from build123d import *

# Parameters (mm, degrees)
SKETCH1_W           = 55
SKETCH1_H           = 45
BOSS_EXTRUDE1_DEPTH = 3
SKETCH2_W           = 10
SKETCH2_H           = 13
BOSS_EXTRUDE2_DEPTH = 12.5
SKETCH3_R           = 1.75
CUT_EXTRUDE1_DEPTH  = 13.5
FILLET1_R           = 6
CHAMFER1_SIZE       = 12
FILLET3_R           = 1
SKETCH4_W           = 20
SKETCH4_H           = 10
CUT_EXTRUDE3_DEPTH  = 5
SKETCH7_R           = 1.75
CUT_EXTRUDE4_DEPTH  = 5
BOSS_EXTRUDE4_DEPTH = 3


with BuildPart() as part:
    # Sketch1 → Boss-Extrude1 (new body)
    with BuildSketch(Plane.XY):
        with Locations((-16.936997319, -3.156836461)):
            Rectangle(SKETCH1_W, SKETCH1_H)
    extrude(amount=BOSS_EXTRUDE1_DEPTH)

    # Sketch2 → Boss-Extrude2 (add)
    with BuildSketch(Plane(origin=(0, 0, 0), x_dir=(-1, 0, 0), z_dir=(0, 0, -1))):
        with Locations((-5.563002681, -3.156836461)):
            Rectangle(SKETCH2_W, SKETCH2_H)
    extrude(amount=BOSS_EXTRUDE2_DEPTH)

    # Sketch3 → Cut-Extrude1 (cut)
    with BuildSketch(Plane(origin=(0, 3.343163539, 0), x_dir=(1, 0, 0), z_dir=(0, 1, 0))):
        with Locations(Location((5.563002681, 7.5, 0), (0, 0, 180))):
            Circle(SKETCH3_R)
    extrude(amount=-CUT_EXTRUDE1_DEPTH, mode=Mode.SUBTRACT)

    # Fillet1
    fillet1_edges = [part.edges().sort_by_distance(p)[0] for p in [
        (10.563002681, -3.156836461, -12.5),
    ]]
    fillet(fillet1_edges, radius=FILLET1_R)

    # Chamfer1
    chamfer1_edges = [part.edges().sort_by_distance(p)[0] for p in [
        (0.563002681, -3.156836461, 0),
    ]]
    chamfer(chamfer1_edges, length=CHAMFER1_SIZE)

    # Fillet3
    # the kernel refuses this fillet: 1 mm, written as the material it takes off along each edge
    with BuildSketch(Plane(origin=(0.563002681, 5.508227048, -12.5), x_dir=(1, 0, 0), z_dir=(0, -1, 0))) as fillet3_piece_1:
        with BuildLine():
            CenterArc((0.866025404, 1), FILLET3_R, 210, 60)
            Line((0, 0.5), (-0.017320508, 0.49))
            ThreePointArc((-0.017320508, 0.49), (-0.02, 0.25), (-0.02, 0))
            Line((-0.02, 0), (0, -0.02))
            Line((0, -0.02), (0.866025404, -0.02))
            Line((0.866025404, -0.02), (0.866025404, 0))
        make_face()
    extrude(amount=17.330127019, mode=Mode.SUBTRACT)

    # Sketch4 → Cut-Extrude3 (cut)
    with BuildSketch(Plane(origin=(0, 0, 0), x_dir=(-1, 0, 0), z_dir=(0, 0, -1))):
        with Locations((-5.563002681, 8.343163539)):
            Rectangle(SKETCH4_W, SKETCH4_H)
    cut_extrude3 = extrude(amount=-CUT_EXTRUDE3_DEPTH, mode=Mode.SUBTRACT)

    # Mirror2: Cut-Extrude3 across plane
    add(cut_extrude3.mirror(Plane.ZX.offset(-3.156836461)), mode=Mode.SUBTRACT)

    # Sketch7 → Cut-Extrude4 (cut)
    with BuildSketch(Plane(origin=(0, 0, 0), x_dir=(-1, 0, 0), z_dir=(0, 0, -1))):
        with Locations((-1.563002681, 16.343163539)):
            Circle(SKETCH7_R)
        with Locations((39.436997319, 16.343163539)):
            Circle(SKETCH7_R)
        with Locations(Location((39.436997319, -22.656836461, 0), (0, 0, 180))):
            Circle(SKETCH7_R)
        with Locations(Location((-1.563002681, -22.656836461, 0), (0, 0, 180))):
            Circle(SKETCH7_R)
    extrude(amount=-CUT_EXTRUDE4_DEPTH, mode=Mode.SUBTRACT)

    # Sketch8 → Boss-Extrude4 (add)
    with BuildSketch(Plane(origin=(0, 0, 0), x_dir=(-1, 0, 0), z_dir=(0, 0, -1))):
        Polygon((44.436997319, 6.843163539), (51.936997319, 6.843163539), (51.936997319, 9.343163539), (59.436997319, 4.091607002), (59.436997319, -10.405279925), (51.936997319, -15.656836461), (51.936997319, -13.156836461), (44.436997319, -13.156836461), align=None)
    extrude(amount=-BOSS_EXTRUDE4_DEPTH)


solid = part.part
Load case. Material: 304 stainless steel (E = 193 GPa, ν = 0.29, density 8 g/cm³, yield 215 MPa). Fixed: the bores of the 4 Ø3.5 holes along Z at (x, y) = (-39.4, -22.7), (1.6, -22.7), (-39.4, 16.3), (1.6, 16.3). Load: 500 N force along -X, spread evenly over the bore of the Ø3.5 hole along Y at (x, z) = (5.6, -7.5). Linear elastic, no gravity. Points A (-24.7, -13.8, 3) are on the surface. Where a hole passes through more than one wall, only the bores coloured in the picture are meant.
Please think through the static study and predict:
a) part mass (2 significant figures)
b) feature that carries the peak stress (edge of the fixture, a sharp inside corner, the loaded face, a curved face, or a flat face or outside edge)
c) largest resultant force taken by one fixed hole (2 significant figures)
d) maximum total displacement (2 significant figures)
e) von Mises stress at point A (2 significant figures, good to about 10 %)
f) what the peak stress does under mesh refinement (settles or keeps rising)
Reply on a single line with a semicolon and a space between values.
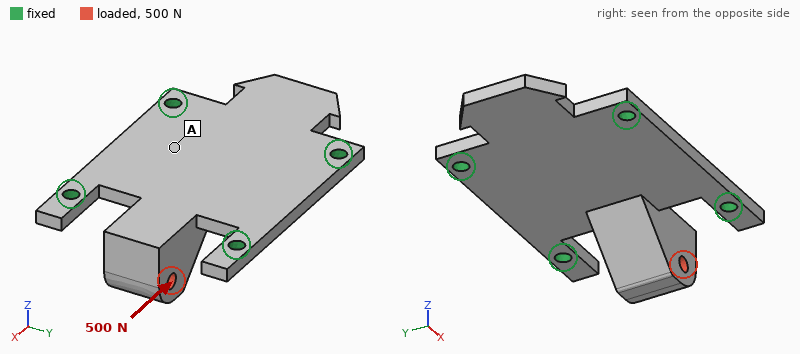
77 g; a sharp inside corner; 200 N; 64 µm; 13 MPa; keeps rising
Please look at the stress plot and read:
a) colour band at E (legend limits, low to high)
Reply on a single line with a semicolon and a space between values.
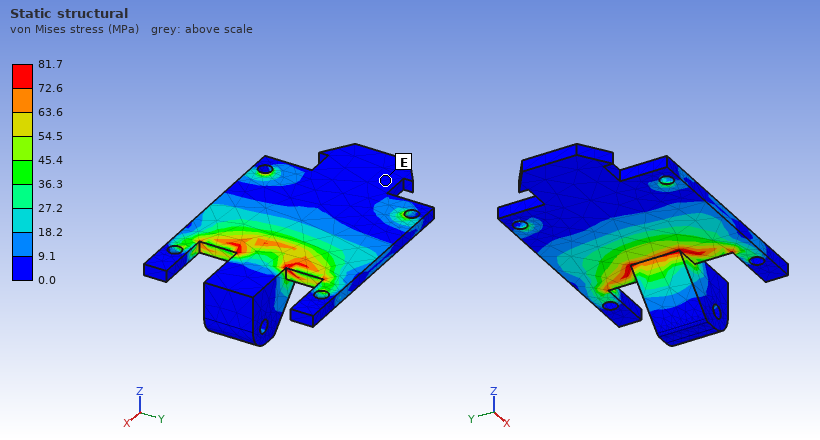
0.0 to 9.1 MPa
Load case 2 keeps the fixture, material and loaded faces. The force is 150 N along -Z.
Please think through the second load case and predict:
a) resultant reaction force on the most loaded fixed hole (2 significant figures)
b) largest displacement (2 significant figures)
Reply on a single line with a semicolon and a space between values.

96 N; 42 µm
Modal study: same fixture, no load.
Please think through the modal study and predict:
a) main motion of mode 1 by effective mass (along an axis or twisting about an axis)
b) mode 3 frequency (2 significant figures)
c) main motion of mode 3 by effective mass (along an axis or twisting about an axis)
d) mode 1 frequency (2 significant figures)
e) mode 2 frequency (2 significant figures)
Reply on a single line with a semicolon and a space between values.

along Z; 5500 Hz; along Z; 2400 Hz; 4200 Hz
